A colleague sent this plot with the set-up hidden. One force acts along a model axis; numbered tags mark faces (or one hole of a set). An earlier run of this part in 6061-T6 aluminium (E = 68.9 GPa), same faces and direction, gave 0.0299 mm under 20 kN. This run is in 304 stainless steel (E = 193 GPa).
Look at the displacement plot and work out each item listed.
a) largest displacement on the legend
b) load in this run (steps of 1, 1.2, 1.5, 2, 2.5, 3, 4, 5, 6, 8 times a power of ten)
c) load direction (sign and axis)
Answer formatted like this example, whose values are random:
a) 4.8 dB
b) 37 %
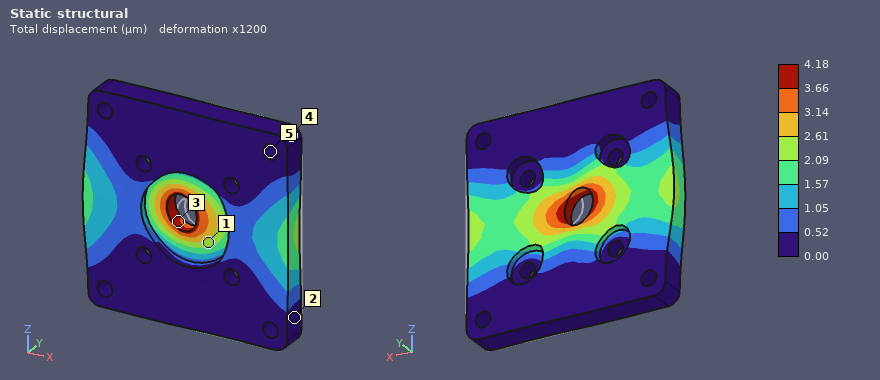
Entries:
a) 4.18 µm
b) 8 kN
c) -X
